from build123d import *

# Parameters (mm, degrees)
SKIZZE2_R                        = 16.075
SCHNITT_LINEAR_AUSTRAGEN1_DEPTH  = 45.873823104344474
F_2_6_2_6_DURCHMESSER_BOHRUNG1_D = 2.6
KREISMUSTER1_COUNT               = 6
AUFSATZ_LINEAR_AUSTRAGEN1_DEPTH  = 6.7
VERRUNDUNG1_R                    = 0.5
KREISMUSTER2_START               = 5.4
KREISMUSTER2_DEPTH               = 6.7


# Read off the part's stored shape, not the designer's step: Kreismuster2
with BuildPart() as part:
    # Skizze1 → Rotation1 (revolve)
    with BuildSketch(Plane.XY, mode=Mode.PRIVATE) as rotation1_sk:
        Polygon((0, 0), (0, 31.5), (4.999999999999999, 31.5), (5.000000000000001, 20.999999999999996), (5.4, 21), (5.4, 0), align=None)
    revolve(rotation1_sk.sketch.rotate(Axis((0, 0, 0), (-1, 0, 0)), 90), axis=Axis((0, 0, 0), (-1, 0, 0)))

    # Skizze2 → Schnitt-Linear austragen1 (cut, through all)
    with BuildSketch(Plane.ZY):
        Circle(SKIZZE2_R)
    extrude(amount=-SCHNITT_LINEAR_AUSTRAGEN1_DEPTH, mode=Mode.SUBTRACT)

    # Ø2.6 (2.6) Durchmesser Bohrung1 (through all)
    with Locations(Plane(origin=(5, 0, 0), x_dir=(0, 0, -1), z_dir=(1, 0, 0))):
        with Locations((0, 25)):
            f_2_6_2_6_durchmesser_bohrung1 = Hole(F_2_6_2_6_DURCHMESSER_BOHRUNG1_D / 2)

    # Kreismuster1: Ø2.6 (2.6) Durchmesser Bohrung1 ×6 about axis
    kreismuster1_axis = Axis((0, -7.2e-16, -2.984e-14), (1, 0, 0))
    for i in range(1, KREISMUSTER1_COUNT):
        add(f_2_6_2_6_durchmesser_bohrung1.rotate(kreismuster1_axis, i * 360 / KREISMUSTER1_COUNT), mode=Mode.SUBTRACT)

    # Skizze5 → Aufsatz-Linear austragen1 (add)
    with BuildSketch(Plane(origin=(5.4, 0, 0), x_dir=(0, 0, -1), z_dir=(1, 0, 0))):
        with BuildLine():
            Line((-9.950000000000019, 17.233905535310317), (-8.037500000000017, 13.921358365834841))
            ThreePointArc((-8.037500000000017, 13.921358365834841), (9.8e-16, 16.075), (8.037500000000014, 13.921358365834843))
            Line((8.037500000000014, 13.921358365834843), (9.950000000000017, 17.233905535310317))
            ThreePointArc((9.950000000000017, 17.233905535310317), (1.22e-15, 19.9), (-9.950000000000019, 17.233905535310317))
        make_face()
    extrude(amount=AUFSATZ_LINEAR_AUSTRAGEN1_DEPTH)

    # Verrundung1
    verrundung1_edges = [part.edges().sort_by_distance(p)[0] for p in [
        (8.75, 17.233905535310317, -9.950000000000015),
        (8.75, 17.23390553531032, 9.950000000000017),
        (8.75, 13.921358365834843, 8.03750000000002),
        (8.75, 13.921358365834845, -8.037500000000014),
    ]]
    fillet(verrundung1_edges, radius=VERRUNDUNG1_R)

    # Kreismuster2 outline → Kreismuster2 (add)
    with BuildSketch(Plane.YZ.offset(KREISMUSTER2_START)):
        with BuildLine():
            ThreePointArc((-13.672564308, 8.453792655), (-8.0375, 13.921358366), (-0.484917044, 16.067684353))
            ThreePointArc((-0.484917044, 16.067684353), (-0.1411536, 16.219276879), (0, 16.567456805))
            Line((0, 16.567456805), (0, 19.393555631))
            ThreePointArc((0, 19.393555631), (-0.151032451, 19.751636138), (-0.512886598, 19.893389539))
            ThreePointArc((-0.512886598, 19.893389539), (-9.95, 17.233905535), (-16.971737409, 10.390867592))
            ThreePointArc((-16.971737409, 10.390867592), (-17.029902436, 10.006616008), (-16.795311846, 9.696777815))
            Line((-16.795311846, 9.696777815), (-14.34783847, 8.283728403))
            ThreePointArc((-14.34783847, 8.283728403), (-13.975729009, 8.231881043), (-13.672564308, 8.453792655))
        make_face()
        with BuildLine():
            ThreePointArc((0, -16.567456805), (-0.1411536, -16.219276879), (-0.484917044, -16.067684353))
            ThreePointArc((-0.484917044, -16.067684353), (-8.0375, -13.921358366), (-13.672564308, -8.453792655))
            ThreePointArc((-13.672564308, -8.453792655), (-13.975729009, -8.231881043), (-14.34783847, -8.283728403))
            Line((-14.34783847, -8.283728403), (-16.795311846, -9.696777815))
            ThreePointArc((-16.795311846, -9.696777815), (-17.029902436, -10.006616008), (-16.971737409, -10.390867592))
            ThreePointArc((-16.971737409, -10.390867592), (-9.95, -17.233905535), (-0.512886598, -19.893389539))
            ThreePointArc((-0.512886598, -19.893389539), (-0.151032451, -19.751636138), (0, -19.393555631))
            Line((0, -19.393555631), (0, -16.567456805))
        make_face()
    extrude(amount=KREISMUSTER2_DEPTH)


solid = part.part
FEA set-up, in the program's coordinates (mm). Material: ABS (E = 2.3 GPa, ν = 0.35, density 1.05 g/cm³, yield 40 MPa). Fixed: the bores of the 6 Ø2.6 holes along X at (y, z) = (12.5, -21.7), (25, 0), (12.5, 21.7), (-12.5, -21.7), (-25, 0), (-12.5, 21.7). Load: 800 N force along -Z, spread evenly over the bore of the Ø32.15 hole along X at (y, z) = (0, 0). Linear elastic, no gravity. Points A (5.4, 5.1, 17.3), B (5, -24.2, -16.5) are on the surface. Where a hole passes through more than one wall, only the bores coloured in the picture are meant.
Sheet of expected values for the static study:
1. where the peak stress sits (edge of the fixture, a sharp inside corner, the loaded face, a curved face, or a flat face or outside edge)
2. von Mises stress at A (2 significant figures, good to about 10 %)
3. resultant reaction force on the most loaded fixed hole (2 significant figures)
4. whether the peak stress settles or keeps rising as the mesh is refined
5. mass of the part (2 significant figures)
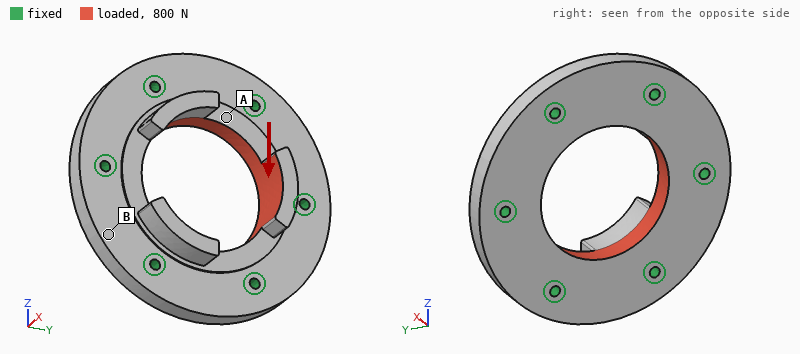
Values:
a sharp inside corner
1.6 MPa
160 N
keeps rising
14 g
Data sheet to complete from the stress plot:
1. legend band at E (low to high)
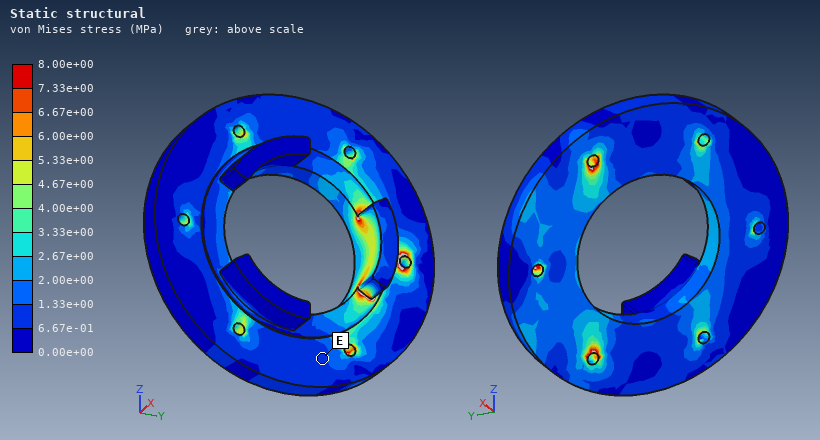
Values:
6.67e-01 to 1.33e+00 MPa
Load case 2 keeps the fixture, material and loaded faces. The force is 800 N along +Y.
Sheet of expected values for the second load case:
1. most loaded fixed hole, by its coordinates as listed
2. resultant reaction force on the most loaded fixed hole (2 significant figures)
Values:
(25, 0)
240 N
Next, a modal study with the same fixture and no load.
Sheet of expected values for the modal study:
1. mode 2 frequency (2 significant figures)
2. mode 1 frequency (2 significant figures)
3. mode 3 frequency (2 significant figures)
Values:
6800 Hz
6500 Hz
7200 Hz
